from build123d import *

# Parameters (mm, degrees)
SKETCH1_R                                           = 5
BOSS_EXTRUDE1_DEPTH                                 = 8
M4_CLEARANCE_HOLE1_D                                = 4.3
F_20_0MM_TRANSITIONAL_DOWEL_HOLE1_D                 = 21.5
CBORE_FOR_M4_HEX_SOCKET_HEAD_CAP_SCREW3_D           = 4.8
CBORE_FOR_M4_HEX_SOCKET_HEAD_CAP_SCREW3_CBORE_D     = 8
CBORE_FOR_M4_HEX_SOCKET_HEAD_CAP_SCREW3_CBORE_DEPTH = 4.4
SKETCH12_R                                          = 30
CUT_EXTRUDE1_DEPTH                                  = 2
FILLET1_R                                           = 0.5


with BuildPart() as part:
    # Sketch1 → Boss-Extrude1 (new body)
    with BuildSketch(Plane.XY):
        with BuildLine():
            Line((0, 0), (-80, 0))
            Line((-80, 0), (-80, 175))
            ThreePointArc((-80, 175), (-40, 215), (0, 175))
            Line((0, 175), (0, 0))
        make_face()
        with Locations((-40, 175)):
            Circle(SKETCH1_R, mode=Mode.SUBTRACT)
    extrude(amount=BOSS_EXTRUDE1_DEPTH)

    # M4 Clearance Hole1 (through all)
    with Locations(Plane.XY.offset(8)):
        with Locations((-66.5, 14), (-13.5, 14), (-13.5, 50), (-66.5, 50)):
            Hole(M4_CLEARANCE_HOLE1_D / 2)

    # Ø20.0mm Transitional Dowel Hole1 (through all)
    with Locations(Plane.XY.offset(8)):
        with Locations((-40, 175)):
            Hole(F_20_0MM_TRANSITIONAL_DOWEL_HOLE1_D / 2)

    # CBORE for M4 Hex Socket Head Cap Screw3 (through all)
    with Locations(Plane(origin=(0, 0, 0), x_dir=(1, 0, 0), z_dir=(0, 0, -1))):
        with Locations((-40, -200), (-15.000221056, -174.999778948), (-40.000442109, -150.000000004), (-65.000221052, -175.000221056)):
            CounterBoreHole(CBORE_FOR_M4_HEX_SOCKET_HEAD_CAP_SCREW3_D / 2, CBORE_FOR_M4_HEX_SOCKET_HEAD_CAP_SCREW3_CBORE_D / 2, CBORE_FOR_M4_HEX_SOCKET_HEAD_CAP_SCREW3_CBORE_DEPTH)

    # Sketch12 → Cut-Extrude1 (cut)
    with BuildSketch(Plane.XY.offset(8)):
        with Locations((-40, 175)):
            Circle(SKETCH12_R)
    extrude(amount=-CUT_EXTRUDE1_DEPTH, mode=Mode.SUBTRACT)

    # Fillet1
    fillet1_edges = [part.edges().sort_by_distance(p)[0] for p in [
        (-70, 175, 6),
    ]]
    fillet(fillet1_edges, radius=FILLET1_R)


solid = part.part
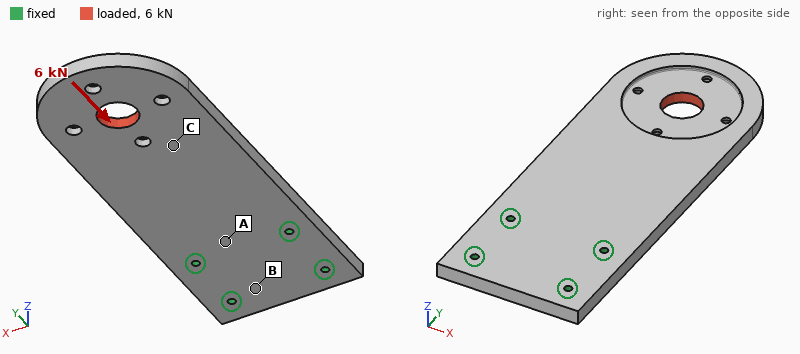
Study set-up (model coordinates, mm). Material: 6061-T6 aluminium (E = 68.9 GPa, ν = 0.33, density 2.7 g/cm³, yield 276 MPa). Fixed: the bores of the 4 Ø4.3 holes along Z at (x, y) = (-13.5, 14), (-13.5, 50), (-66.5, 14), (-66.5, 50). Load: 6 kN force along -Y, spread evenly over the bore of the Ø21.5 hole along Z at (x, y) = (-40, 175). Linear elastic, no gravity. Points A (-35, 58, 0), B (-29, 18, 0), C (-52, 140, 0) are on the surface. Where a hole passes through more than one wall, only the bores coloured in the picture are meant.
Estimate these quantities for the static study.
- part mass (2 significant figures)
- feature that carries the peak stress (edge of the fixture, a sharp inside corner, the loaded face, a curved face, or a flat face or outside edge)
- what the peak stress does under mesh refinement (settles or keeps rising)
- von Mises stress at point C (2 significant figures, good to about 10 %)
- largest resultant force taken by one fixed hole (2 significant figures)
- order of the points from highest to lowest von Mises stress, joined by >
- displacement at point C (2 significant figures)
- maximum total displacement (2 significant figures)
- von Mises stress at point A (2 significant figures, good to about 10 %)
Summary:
330 g
a sharp inside corner
keeps rising
20 MPa
2.3 kN
C > A > B
0.11 mm
0.32 mm
11 MPa
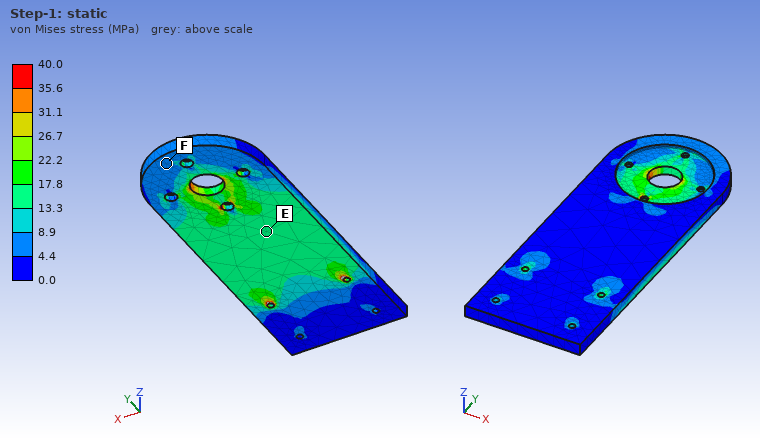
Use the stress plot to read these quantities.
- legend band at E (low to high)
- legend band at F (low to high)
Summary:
13.3 to 17.8 MPa
4.4 to 8.9 MPa
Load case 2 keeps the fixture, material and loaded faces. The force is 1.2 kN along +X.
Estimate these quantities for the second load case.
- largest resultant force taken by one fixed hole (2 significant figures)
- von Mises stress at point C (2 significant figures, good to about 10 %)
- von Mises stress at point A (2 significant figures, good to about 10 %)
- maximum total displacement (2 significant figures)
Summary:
2.3 kN
5.0 MPa
3.6 MPa
72 µm
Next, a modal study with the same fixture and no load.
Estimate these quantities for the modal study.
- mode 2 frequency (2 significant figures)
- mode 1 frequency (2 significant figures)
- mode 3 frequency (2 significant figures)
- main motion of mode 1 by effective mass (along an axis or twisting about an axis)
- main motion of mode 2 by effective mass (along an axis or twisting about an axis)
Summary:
1100 Hz
280 Hz
1500 Hz
along Z
twisting about Y
